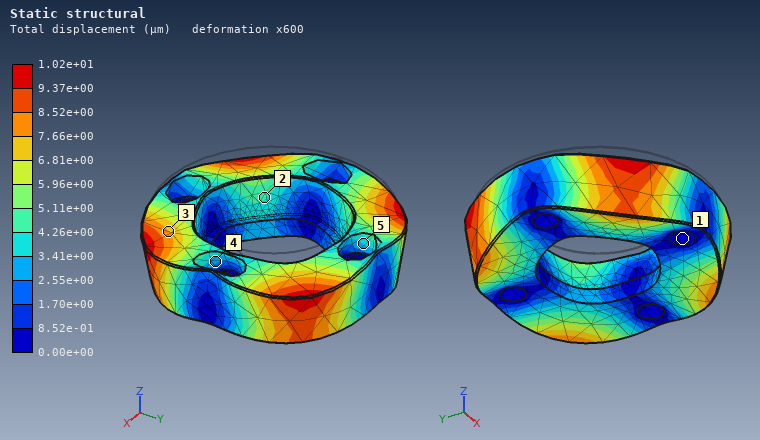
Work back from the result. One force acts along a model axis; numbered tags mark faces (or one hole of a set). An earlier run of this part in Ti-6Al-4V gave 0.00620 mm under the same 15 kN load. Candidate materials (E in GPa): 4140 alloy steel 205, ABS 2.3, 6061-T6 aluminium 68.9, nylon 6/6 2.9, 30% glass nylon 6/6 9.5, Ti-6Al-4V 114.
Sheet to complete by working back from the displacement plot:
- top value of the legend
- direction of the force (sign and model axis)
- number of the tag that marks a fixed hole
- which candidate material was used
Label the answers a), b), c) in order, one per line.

a) 1.02e+01 µm
b) -Z
c) 1
d) 6061-T6 aluminium
